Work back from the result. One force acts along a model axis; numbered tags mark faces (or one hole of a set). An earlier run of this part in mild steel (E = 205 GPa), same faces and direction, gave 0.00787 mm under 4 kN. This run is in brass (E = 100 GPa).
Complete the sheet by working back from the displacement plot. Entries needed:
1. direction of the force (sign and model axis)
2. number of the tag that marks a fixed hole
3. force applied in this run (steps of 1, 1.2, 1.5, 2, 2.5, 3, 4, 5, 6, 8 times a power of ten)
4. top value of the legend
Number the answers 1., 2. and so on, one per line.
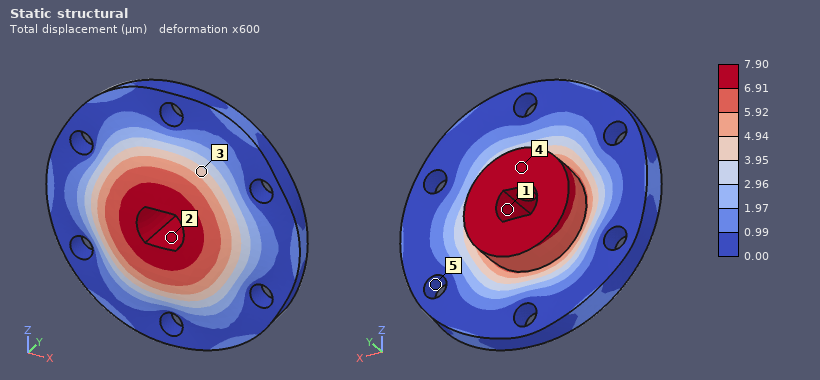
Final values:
1. -Y
2. 5
3. 2 kN
4. 7.90 µm
